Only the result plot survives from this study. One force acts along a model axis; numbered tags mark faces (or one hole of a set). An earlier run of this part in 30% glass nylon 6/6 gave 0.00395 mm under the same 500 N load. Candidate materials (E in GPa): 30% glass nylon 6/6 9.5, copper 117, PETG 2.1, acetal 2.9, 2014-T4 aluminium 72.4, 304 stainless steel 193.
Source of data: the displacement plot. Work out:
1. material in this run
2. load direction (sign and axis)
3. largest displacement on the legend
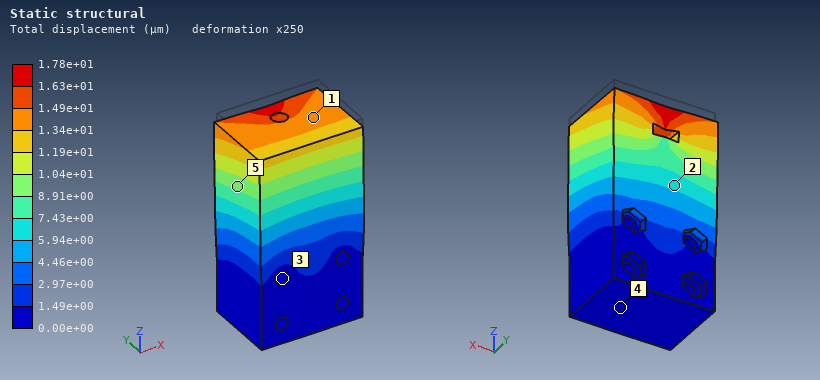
PETG
-Z
1.78e+01 µm
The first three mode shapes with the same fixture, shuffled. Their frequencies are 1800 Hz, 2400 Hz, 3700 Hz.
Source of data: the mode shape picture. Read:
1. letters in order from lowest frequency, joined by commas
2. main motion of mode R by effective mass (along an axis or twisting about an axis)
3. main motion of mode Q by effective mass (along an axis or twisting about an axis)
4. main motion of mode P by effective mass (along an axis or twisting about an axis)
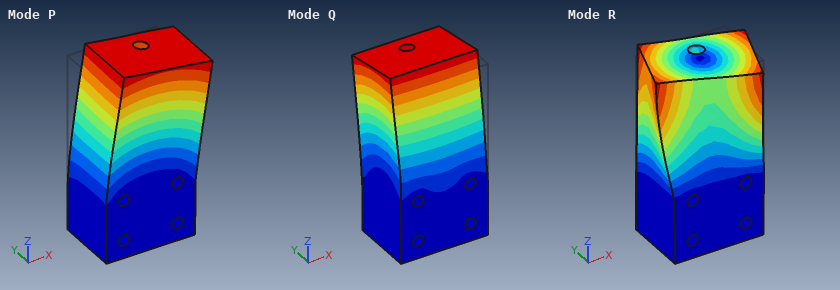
Q, P, R
twisting about Z
along Y
along X
